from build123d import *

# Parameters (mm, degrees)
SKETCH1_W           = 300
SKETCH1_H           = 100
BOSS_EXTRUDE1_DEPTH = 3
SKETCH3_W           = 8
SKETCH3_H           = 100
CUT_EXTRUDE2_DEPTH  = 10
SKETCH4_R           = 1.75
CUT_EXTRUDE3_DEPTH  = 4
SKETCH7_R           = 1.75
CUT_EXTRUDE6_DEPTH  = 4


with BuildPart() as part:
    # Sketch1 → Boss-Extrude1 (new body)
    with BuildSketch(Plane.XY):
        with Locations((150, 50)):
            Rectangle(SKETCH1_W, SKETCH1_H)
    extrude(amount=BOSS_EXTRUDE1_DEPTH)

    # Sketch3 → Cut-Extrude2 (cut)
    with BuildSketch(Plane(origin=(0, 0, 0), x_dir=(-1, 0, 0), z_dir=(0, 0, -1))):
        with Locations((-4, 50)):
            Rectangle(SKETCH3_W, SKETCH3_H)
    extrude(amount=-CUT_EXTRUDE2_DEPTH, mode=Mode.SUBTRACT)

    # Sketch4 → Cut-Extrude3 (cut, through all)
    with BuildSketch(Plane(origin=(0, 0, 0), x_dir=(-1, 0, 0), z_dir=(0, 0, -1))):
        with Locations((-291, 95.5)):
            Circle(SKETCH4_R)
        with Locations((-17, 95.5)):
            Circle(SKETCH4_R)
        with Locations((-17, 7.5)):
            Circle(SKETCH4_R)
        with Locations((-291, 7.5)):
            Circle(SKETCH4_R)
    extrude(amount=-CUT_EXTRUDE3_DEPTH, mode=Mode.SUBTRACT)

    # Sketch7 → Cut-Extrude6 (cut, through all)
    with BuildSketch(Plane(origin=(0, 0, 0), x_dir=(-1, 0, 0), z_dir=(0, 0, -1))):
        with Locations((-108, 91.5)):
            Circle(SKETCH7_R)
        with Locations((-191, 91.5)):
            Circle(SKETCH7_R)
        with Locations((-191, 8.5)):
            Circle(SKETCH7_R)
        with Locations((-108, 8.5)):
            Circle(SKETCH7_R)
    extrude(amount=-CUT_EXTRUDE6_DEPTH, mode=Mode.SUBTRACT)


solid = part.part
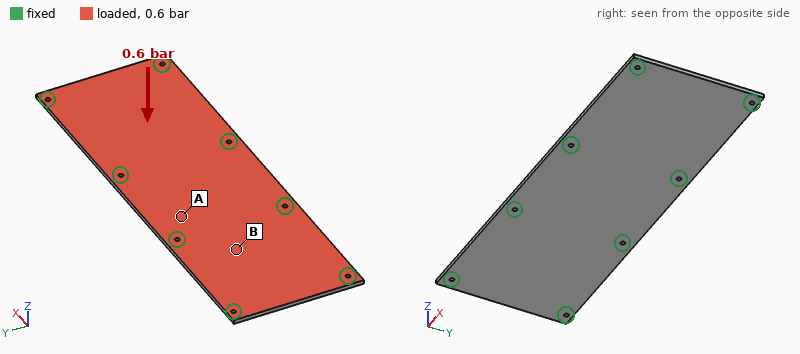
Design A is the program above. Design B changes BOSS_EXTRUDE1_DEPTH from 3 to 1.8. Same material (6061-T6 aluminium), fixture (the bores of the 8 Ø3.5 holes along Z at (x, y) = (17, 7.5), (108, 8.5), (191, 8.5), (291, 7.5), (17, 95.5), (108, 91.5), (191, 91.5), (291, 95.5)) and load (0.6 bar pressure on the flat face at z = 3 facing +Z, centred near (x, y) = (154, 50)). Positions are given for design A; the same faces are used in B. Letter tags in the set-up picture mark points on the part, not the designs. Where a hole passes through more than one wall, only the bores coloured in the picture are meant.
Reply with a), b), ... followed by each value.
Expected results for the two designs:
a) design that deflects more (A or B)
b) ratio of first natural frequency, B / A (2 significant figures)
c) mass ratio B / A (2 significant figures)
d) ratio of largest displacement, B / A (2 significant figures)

a) B
b) 0.61
c) 0.60
d) 4.4
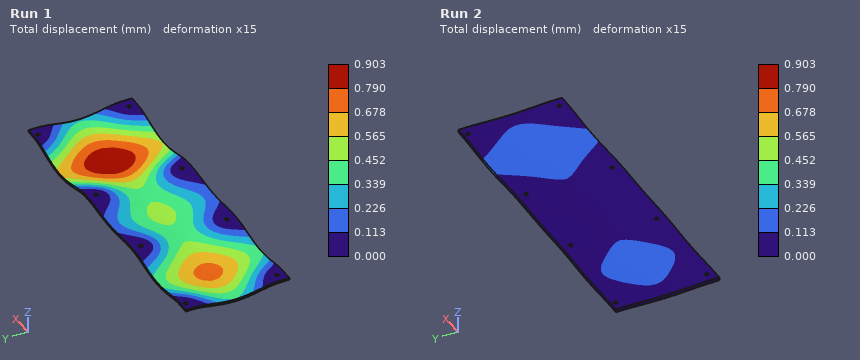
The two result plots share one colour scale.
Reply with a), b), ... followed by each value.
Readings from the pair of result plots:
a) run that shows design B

a) Run 1
